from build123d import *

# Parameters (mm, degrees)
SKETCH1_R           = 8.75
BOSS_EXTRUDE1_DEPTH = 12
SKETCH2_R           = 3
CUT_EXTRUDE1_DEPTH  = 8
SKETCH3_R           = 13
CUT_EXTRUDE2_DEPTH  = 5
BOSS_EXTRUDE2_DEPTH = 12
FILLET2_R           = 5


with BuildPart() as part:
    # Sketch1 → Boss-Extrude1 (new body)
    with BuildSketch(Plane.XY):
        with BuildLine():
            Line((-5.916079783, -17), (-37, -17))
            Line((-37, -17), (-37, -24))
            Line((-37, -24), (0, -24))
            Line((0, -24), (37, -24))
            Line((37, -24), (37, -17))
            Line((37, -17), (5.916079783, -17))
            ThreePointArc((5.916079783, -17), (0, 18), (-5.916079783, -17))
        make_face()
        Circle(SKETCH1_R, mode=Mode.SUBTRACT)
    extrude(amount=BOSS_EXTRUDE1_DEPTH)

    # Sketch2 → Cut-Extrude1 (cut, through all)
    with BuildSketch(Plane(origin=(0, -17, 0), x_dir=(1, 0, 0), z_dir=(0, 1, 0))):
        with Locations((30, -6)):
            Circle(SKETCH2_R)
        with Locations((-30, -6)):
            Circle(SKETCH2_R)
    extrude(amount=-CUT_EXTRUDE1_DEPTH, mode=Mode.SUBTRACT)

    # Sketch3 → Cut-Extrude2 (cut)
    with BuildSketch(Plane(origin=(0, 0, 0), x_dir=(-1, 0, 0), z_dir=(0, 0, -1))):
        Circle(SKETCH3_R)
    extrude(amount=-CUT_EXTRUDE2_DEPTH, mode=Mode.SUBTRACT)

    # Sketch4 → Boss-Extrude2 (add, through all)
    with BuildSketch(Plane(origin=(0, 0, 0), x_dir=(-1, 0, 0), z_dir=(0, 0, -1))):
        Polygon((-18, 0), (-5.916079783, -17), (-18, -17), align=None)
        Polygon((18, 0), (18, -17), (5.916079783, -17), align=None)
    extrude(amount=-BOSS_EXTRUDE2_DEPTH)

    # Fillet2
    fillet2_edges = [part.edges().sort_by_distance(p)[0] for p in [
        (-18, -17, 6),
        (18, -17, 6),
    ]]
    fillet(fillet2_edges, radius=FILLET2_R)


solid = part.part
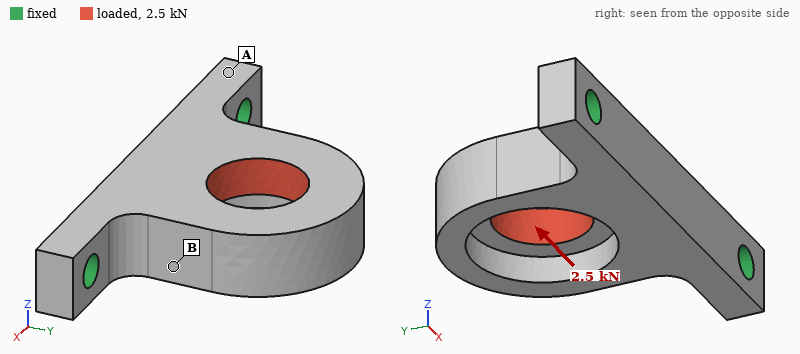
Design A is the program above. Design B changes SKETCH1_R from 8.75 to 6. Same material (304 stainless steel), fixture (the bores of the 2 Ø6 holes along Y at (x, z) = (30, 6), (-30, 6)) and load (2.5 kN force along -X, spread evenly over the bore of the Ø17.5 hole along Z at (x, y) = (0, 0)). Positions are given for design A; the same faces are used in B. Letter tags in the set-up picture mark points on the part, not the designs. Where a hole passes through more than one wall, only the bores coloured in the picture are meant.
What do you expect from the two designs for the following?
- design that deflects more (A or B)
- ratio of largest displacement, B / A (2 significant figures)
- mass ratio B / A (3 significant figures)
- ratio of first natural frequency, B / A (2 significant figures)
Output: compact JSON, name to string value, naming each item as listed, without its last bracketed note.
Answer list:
{"design that deflects more": "A", "ratio of largest displacement, B / A": "0.82", "mass ratio B / A": "1.06", "ratio of first natural frequency, B / A": "0.96"}
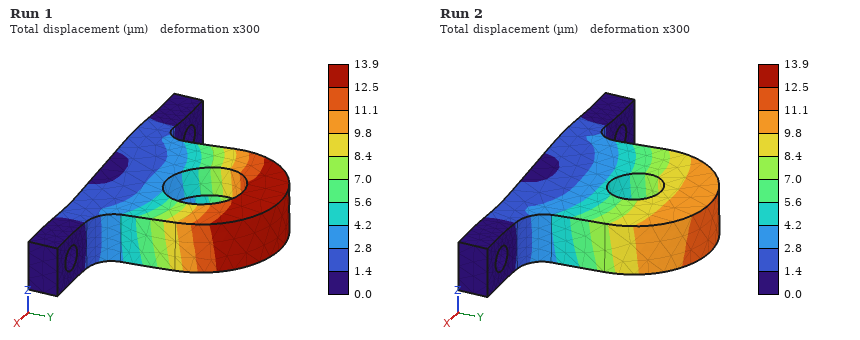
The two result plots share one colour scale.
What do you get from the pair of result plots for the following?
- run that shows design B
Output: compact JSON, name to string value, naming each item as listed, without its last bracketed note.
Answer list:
{"run that shows design B": "Run 2"}
